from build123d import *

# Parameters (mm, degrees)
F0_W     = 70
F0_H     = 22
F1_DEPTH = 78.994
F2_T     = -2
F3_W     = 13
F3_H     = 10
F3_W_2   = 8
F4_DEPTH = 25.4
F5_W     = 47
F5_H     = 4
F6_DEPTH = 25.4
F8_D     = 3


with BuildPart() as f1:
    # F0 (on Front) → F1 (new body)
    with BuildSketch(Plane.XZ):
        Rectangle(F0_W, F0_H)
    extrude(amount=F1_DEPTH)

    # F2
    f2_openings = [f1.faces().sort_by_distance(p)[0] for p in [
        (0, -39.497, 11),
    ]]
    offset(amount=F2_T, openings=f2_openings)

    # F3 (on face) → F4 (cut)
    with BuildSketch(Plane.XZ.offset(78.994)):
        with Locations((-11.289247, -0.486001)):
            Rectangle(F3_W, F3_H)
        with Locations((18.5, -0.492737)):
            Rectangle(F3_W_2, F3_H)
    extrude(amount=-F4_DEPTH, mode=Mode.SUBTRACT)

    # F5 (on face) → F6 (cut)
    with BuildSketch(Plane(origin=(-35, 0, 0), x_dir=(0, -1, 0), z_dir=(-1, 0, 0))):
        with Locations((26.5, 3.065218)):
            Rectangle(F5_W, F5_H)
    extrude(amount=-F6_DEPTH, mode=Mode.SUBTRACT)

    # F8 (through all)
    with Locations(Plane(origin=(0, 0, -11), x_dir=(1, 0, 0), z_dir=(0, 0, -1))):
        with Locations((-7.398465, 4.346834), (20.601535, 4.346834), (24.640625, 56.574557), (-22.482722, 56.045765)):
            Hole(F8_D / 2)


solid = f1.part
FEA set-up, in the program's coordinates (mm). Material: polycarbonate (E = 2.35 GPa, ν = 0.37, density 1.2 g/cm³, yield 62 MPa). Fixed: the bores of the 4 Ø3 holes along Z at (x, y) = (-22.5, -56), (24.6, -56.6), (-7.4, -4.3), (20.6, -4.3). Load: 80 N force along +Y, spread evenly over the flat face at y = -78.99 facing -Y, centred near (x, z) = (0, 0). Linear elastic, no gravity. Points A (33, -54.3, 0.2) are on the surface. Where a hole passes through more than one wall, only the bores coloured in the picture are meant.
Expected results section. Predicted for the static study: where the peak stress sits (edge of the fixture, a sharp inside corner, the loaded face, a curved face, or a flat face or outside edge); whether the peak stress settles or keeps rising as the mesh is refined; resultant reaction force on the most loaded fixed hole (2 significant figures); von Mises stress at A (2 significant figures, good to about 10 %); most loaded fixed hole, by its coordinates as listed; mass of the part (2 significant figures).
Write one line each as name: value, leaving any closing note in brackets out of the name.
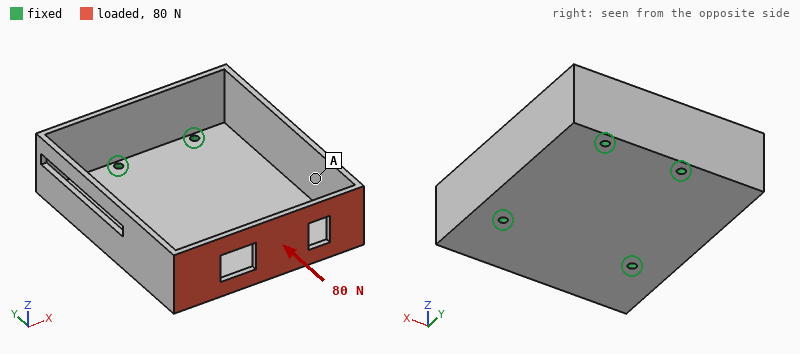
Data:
where the peak stress sits: edge of the fixture
whether the peak stress settles or keeps rising as the mesh is refined: keeps rising
resultant reaction force on the most loaded fixed hole: 33 N
von Mises stress at A: 1.2 MPa
most loaded fixed hole, by its coordinates as listed: (-22.5, -56)
mass of the part: 26 g
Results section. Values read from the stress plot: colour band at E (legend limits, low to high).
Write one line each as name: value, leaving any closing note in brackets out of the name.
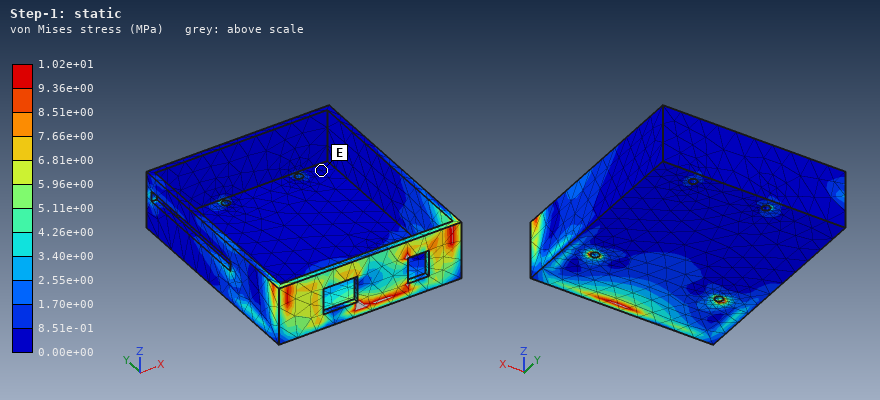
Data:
colour band at E: 0.00e+00 to 8.51e-01 MPa
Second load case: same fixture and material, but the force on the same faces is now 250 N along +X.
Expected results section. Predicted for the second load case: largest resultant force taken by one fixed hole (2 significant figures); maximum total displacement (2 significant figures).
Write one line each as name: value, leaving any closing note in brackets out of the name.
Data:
largest resultant force taken by one fixed hole: 180 N
maximum total displacement: 0.99 mm
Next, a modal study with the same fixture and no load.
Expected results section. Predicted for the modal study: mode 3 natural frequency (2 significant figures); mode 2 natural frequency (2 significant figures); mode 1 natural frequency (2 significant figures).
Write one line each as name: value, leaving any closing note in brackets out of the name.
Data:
mode 3 natural frequency: 810 Hz
mode 2 natural frequency: 790 Hz
mode 1 natural frequency: 660 Hz
